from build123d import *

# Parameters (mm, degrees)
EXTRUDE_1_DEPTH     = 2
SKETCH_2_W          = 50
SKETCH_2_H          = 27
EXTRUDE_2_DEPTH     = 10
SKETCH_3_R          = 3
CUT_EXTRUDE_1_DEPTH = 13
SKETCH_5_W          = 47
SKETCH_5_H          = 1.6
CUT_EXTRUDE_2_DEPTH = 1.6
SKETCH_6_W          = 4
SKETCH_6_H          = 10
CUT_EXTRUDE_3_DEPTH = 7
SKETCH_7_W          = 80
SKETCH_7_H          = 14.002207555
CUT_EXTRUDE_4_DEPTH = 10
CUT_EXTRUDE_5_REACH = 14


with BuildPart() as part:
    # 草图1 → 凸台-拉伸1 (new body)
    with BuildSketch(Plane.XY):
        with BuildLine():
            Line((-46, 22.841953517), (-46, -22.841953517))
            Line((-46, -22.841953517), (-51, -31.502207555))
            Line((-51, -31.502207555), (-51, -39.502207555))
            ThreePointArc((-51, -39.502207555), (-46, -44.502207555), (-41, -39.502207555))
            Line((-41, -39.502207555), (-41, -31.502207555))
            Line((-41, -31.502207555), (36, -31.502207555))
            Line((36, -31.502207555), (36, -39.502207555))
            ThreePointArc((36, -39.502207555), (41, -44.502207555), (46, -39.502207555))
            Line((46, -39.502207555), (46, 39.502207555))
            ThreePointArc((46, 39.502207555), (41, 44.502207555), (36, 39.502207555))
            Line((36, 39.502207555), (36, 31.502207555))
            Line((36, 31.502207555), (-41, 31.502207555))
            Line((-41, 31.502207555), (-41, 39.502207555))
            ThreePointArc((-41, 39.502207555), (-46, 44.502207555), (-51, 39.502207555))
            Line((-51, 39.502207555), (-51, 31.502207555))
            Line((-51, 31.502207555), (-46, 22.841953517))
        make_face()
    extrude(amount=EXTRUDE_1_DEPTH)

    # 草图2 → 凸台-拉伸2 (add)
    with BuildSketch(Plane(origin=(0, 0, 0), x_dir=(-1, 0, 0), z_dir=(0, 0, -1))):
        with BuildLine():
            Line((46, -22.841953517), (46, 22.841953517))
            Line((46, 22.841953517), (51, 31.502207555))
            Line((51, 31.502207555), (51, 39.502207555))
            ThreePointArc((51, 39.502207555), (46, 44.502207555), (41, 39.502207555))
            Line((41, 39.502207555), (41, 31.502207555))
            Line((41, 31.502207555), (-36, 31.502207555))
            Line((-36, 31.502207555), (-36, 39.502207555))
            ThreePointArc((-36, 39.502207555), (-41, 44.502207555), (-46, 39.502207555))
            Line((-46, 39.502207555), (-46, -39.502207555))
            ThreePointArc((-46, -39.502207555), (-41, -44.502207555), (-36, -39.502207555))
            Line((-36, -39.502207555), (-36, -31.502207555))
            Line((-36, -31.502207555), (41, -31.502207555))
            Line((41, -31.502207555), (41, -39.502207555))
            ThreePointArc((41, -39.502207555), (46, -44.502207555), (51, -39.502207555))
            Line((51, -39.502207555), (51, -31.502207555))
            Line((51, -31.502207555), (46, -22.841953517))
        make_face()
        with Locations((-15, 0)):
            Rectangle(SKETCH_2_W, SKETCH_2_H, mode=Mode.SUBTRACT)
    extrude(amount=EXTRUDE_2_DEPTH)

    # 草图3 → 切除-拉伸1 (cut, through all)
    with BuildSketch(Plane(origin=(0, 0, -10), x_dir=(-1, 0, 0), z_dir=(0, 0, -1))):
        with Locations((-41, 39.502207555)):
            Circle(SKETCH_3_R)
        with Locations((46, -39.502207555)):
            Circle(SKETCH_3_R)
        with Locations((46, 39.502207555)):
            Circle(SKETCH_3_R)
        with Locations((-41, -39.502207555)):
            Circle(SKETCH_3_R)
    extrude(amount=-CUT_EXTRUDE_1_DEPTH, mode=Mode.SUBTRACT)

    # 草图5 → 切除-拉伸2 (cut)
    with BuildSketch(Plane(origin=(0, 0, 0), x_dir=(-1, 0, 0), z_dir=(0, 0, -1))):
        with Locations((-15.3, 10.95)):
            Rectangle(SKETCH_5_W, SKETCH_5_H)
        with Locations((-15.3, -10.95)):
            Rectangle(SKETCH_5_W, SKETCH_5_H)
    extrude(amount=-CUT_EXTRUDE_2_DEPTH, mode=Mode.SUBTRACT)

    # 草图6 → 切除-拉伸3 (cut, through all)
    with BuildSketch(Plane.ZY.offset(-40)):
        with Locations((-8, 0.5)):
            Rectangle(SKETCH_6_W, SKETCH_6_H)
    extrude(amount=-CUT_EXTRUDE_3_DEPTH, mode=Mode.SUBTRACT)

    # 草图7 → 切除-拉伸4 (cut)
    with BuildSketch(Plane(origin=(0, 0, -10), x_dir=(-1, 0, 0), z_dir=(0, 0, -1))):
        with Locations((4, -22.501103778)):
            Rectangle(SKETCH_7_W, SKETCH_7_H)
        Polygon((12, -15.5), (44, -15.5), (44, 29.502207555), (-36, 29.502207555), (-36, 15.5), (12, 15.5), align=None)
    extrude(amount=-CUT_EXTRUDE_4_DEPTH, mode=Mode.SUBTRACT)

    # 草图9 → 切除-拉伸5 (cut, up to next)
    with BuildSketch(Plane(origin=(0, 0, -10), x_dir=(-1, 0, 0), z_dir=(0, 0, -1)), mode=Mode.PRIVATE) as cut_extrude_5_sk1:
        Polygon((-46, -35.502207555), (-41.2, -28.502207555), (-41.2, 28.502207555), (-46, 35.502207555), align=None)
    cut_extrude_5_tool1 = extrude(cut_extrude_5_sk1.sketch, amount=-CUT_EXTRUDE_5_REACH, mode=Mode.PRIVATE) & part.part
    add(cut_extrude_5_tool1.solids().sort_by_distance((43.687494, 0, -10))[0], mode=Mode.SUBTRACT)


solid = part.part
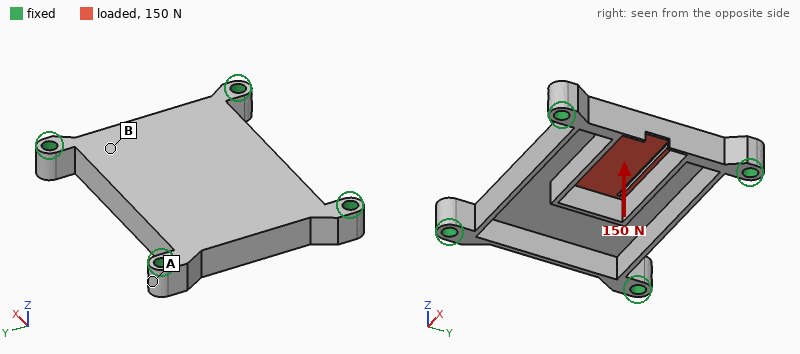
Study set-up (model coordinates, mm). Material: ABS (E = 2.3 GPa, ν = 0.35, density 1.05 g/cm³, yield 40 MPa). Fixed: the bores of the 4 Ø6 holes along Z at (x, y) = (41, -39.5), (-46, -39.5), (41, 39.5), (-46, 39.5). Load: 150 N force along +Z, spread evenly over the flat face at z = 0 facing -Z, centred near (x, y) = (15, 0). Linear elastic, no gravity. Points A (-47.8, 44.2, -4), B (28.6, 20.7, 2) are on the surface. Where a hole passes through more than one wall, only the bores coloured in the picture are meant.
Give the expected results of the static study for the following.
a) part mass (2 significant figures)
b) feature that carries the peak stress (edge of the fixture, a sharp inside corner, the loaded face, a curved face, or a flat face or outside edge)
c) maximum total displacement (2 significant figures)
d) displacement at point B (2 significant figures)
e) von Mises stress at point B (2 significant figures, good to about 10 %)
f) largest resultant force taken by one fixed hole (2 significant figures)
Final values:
26 g
a flat face or outside edge
0.78 mm
0.15 mm
2.0 MPa
74 N
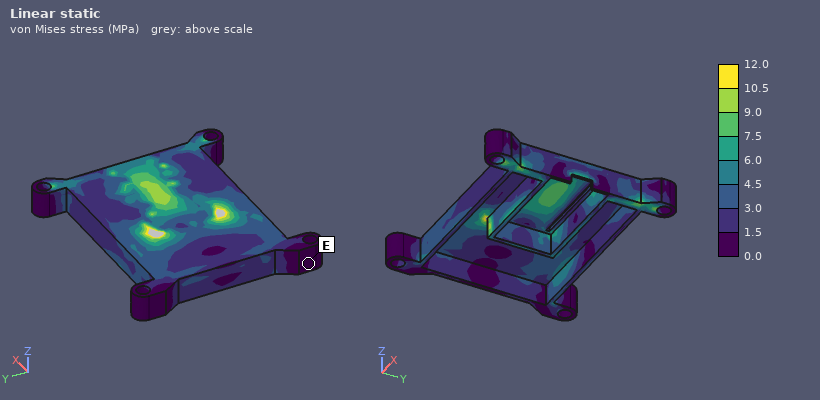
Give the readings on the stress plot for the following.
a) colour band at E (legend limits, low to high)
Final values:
0.0 to 1.5 MPa
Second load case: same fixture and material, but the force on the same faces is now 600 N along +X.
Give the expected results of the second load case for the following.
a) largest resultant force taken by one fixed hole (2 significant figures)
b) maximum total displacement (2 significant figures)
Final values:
170 N
0.17 mm
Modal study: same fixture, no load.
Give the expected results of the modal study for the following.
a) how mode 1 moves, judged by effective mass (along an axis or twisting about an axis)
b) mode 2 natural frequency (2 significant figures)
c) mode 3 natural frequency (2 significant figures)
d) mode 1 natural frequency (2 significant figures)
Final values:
along Z
1400 Hz
1900 Hz
800 Hz
